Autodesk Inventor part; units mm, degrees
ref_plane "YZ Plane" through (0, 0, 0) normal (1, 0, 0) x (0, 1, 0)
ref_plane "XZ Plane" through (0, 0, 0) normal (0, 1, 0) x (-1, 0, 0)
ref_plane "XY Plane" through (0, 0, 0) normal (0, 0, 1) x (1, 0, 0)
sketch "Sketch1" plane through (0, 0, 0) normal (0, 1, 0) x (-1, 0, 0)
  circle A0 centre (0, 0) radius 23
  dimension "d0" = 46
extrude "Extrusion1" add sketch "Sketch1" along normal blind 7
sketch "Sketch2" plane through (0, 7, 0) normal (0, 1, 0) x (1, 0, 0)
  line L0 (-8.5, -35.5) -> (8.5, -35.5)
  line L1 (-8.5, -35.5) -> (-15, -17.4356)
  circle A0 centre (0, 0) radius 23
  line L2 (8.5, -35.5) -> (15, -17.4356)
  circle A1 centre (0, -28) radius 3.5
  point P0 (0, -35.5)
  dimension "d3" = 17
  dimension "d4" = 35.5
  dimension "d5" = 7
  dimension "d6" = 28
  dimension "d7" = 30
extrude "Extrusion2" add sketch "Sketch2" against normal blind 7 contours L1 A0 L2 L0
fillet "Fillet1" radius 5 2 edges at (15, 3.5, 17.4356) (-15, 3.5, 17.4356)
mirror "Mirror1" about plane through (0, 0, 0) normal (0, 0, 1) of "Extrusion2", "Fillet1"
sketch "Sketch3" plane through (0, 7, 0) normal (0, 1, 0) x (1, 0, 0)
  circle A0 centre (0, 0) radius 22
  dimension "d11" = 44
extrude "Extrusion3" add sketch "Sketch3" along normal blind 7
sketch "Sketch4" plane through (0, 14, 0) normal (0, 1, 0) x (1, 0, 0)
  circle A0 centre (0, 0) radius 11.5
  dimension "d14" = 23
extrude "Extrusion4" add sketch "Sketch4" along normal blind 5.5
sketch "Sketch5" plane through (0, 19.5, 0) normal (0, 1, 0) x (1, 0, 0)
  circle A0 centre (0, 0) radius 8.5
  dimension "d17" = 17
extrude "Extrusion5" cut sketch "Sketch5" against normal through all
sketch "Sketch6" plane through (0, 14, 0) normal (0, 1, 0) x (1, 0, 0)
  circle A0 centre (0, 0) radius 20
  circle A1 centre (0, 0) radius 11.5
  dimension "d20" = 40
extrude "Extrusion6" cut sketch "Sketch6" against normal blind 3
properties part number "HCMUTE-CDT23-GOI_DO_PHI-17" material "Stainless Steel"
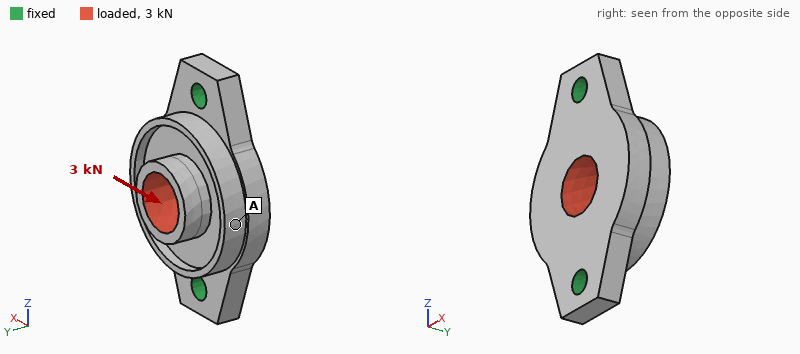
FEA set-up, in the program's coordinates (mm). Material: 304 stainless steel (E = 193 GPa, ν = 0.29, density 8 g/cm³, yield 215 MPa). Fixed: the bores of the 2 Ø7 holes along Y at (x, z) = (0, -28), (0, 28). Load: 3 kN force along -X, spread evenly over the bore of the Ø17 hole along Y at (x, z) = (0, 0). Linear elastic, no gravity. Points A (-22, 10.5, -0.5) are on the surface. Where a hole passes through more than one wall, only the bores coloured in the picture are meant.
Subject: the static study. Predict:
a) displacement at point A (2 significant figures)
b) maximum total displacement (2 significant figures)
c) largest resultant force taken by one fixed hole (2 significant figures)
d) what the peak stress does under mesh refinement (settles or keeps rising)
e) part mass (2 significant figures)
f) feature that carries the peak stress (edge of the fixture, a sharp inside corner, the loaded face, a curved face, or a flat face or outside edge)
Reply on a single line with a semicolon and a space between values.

10 µm; 11 µm; 1.5 kN; keeps rising; 170 g; edge of the fixture
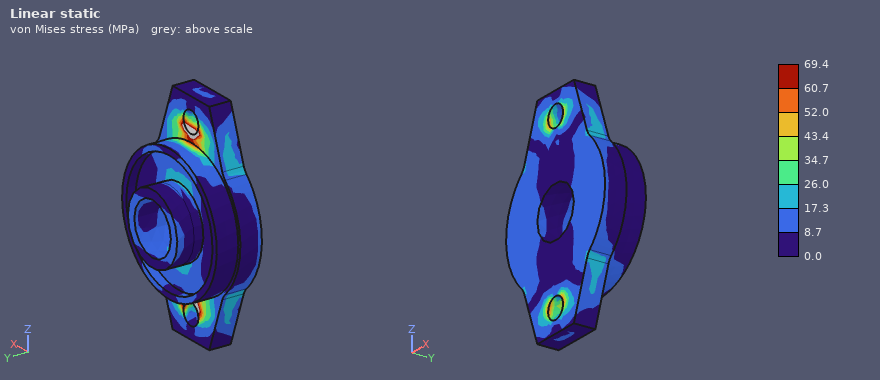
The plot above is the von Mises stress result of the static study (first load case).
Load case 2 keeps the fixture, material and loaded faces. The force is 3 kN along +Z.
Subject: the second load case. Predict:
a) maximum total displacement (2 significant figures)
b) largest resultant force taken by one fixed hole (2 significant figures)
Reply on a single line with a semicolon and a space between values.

2.7 µm; 1.5 kN
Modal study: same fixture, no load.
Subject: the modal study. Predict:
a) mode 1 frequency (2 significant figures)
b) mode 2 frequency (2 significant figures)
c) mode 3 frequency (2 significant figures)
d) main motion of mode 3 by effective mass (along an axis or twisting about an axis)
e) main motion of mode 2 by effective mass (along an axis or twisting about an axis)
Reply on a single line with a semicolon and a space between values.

6800 Hz; 9300 Hz; 18 kHz; along X; along Y
